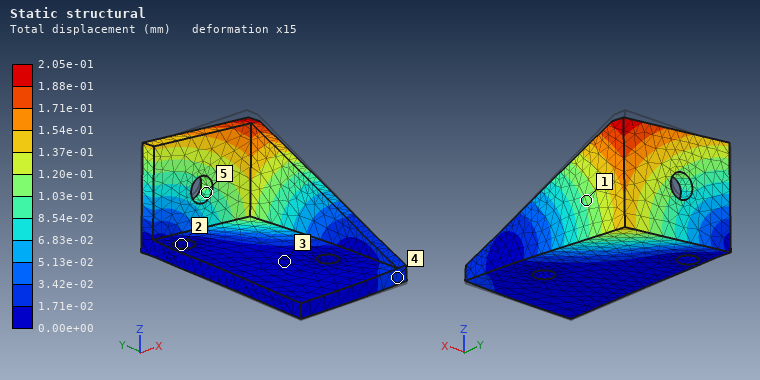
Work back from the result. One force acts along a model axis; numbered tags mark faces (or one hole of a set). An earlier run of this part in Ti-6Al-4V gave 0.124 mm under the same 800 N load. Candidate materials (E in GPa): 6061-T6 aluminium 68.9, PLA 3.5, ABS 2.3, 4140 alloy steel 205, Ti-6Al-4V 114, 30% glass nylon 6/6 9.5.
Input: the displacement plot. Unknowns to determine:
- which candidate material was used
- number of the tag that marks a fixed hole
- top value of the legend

6061-T6 aluminium
2
2.05e-01 mm
